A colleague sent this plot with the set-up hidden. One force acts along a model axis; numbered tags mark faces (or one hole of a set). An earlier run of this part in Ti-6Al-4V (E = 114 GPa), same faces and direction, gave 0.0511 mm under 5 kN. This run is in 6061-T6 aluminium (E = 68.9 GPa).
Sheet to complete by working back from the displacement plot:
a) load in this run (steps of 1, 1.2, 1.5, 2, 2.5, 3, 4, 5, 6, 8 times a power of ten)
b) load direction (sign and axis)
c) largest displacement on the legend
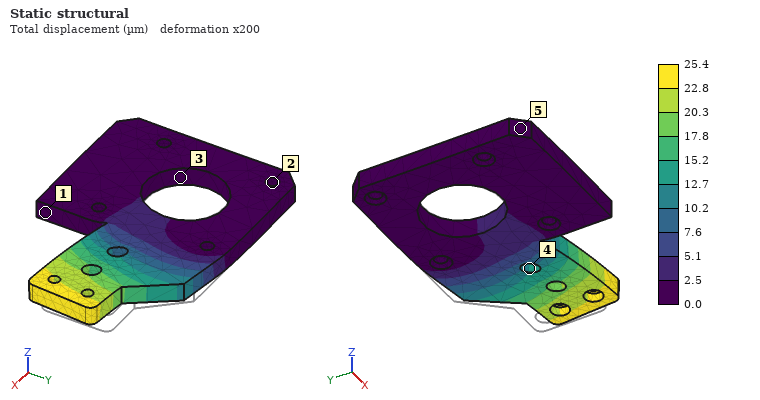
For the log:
1.5 kN
-Y
25.4 µm
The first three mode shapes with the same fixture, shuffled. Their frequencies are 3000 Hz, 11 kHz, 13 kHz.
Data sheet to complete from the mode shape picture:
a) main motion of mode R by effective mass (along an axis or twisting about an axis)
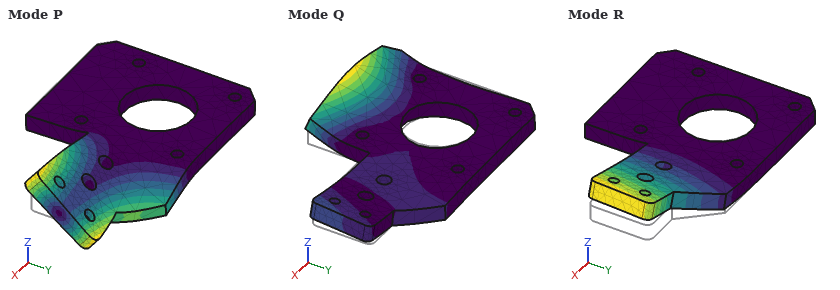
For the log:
along Z
